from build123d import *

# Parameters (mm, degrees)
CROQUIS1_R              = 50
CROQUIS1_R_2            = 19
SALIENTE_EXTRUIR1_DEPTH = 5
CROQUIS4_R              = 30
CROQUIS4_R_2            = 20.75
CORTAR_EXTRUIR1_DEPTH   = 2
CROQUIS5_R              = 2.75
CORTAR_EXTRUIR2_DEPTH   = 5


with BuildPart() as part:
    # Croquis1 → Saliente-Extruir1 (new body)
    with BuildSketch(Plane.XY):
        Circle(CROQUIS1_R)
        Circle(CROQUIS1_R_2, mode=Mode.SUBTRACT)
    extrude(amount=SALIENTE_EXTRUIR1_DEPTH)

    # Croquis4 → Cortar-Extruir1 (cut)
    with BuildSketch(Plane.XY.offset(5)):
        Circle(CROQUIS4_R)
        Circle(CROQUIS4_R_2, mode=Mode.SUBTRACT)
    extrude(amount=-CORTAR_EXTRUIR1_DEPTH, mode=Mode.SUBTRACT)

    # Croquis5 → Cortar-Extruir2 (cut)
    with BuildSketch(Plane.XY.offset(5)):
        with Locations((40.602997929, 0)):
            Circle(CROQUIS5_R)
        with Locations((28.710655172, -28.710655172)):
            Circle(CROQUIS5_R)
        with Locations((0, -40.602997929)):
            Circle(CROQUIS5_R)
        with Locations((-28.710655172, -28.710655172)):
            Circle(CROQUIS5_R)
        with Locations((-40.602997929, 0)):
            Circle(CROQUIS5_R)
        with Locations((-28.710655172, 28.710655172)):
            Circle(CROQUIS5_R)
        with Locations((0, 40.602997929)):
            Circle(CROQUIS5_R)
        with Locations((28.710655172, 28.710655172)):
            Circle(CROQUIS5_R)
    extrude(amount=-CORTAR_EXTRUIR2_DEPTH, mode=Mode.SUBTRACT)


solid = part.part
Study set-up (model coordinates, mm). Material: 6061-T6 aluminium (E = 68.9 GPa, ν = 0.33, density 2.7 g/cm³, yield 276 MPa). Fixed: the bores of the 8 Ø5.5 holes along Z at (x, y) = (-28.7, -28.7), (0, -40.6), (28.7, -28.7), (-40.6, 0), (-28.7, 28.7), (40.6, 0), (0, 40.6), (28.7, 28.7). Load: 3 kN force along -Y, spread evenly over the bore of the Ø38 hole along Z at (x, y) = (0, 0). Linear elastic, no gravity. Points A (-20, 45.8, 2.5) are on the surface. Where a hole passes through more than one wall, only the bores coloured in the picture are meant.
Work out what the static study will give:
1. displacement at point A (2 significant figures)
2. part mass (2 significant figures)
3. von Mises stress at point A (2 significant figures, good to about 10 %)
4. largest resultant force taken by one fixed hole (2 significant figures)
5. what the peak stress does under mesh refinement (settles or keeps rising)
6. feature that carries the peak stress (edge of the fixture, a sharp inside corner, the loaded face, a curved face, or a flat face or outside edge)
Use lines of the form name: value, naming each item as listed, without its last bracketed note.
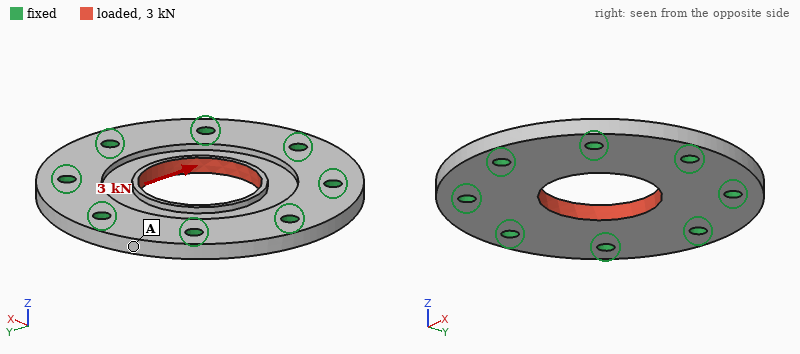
displacement at point A: 0.95 µm
part mass: 80 g
von Mises stress at point A: 2.7 MPa
largest resultant force taken by one fixed hole: 570 N
what the peak stress does under mesh refinement: keeps rising
feature that carries the peak stress: edge of the fixture
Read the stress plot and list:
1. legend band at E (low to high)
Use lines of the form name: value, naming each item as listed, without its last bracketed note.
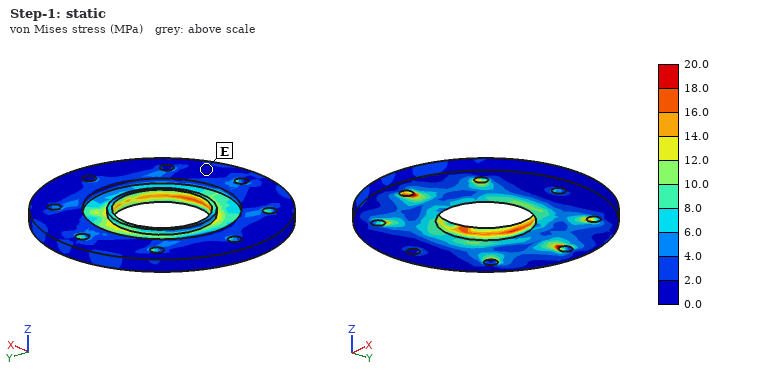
legend band at E: 0.0 to 2.0 MPa
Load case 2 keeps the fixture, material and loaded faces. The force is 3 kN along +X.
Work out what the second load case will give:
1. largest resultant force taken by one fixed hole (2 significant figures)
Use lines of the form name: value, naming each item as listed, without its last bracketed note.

largest resultant force taken by one fixed hole: 570 N
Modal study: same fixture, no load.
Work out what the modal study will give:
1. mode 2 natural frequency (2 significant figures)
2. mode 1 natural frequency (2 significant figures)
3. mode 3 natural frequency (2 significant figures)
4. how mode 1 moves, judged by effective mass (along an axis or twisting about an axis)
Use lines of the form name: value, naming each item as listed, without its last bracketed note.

mode 2 natural frequency: 13 kHz
mode 1 natural frequency: 11 kHz
mode 3 natural frequency: 13 kHz
how mode 1 moves, judged by effective mass: along Z
